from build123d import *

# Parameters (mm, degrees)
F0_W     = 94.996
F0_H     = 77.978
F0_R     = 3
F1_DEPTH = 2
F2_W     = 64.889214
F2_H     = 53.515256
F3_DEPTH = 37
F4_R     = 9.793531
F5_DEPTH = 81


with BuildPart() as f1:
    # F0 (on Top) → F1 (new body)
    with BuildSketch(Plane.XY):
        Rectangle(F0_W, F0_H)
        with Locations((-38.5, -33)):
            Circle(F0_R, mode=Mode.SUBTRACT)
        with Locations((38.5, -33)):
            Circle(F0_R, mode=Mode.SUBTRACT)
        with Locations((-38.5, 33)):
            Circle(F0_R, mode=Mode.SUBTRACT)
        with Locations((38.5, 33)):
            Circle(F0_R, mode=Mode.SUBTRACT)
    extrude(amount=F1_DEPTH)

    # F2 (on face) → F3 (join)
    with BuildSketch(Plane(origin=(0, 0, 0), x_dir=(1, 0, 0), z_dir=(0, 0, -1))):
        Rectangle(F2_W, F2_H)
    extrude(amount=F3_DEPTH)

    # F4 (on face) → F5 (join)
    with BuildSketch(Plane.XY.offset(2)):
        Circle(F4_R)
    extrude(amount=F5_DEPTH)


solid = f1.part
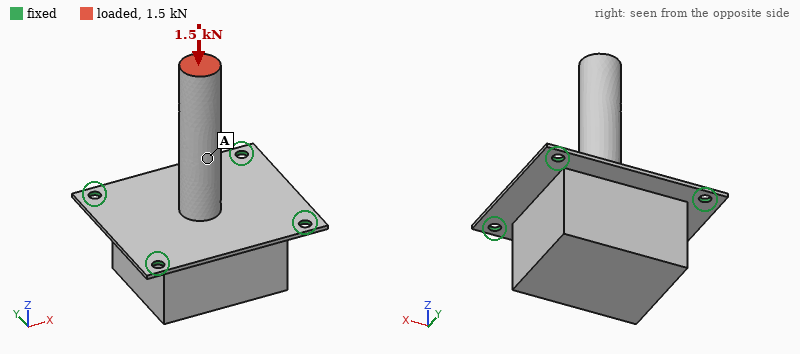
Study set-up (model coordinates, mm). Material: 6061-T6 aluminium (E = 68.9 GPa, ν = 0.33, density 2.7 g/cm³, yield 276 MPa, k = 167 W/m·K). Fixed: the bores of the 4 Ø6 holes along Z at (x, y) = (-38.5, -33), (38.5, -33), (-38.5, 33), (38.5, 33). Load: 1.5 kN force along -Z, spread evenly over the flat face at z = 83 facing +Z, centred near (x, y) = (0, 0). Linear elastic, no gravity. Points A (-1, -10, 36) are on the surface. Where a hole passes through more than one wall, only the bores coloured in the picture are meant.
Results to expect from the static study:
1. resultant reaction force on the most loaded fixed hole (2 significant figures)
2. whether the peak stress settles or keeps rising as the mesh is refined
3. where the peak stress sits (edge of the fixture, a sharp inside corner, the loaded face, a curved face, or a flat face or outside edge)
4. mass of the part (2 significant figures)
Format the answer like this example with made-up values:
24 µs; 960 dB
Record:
430 N; keeps rising; edge of the fixture; 450 g
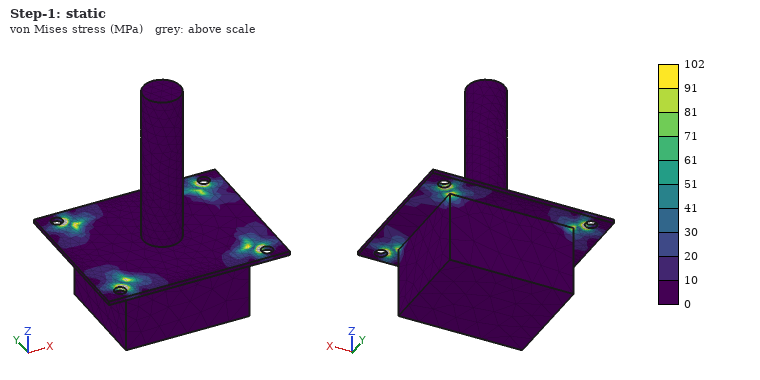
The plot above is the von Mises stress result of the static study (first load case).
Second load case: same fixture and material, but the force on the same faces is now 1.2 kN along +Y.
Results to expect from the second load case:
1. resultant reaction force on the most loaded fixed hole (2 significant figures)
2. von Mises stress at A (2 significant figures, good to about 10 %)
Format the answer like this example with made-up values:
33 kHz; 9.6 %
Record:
910 N; 75 MPa
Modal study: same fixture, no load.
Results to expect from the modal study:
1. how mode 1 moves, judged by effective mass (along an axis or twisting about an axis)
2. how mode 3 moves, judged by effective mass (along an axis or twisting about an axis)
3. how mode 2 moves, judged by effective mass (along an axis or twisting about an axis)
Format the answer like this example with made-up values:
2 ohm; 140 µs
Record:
twisting about X; along Z; twisting about Y
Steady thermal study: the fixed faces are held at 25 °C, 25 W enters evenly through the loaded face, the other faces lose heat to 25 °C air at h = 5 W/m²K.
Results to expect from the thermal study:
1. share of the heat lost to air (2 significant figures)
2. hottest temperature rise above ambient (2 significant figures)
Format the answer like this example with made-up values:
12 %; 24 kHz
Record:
7.8 %; 53 K
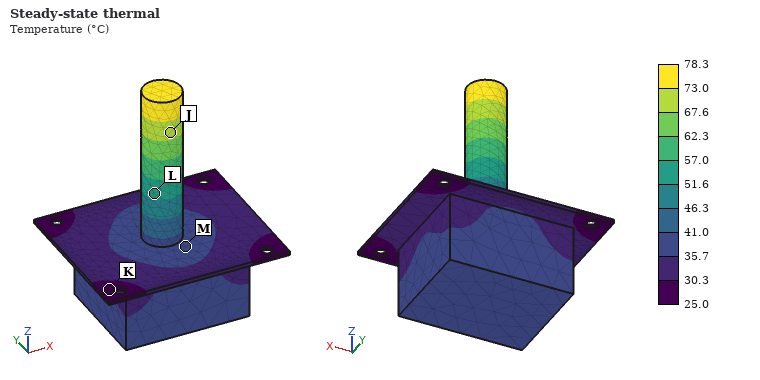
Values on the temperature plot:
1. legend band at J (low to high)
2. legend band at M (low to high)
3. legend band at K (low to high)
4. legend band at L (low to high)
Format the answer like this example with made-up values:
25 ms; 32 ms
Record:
67.6 to 73.0 °C; 35.7 to 41.0 °C; 25.0 to 30.3 °C; 51.6 to 57.0 °C
